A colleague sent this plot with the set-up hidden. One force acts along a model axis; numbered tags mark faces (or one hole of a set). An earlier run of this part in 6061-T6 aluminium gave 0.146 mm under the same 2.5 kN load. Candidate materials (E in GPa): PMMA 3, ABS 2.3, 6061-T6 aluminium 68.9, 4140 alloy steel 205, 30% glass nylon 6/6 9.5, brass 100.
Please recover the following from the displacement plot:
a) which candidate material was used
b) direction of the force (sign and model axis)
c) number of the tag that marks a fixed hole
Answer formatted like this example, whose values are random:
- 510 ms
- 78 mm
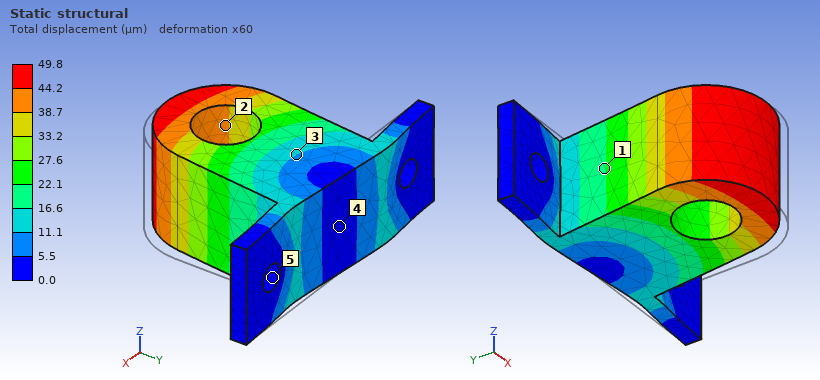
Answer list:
- 4140 alloy steel
- -X
- 5
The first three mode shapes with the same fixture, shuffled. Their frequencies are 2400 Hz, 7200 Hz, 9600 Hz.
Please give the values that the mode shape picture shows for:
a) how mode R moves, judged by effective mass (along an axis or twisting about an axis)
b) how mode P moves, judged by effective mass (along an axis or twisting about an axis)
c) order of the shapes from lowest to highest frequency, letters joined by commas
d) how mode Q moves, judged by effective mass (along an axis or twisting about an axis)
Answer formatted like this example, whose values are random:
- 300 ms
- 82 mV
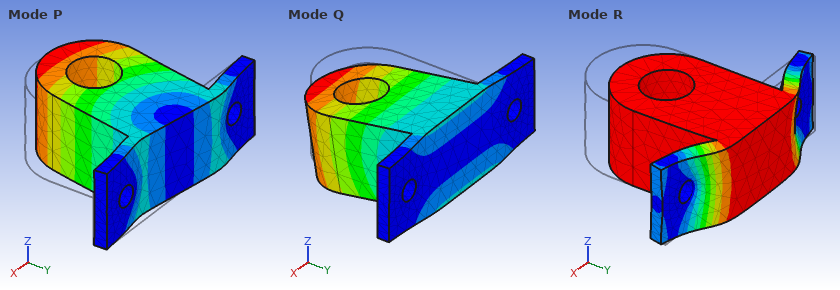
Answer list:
- along Y
- along X
- Q, P, R
- along Z
